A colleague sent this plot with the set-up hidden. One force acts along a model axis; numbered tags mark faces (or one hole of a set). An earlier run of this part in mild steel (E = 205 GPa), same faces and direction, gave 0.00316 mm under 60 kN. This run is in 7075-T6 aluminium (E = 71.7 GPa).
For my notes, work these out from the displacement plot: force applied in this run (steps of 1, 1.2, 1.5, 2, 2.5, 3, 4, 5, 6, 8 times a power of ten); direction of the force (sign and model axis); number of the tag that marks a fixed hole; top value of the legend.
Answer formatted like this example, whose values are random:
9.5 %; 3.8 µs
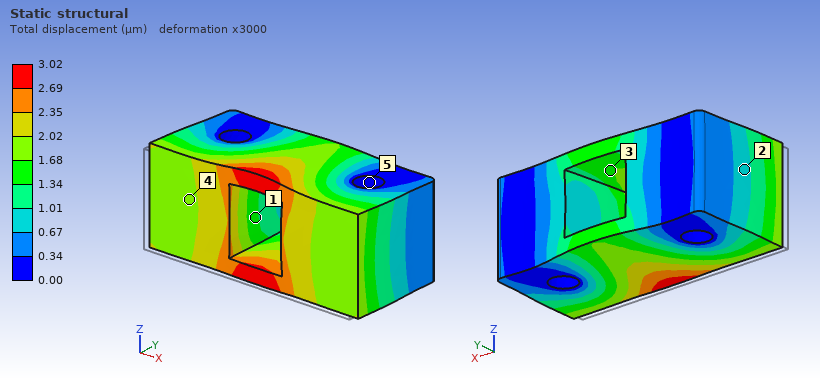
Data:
20 kN; +Y; 5; 3.02 µm
